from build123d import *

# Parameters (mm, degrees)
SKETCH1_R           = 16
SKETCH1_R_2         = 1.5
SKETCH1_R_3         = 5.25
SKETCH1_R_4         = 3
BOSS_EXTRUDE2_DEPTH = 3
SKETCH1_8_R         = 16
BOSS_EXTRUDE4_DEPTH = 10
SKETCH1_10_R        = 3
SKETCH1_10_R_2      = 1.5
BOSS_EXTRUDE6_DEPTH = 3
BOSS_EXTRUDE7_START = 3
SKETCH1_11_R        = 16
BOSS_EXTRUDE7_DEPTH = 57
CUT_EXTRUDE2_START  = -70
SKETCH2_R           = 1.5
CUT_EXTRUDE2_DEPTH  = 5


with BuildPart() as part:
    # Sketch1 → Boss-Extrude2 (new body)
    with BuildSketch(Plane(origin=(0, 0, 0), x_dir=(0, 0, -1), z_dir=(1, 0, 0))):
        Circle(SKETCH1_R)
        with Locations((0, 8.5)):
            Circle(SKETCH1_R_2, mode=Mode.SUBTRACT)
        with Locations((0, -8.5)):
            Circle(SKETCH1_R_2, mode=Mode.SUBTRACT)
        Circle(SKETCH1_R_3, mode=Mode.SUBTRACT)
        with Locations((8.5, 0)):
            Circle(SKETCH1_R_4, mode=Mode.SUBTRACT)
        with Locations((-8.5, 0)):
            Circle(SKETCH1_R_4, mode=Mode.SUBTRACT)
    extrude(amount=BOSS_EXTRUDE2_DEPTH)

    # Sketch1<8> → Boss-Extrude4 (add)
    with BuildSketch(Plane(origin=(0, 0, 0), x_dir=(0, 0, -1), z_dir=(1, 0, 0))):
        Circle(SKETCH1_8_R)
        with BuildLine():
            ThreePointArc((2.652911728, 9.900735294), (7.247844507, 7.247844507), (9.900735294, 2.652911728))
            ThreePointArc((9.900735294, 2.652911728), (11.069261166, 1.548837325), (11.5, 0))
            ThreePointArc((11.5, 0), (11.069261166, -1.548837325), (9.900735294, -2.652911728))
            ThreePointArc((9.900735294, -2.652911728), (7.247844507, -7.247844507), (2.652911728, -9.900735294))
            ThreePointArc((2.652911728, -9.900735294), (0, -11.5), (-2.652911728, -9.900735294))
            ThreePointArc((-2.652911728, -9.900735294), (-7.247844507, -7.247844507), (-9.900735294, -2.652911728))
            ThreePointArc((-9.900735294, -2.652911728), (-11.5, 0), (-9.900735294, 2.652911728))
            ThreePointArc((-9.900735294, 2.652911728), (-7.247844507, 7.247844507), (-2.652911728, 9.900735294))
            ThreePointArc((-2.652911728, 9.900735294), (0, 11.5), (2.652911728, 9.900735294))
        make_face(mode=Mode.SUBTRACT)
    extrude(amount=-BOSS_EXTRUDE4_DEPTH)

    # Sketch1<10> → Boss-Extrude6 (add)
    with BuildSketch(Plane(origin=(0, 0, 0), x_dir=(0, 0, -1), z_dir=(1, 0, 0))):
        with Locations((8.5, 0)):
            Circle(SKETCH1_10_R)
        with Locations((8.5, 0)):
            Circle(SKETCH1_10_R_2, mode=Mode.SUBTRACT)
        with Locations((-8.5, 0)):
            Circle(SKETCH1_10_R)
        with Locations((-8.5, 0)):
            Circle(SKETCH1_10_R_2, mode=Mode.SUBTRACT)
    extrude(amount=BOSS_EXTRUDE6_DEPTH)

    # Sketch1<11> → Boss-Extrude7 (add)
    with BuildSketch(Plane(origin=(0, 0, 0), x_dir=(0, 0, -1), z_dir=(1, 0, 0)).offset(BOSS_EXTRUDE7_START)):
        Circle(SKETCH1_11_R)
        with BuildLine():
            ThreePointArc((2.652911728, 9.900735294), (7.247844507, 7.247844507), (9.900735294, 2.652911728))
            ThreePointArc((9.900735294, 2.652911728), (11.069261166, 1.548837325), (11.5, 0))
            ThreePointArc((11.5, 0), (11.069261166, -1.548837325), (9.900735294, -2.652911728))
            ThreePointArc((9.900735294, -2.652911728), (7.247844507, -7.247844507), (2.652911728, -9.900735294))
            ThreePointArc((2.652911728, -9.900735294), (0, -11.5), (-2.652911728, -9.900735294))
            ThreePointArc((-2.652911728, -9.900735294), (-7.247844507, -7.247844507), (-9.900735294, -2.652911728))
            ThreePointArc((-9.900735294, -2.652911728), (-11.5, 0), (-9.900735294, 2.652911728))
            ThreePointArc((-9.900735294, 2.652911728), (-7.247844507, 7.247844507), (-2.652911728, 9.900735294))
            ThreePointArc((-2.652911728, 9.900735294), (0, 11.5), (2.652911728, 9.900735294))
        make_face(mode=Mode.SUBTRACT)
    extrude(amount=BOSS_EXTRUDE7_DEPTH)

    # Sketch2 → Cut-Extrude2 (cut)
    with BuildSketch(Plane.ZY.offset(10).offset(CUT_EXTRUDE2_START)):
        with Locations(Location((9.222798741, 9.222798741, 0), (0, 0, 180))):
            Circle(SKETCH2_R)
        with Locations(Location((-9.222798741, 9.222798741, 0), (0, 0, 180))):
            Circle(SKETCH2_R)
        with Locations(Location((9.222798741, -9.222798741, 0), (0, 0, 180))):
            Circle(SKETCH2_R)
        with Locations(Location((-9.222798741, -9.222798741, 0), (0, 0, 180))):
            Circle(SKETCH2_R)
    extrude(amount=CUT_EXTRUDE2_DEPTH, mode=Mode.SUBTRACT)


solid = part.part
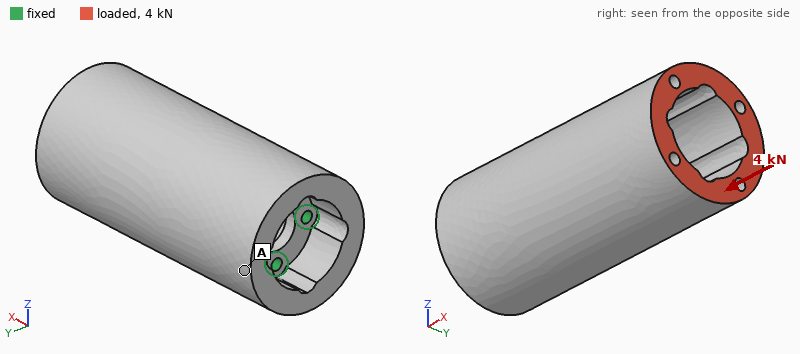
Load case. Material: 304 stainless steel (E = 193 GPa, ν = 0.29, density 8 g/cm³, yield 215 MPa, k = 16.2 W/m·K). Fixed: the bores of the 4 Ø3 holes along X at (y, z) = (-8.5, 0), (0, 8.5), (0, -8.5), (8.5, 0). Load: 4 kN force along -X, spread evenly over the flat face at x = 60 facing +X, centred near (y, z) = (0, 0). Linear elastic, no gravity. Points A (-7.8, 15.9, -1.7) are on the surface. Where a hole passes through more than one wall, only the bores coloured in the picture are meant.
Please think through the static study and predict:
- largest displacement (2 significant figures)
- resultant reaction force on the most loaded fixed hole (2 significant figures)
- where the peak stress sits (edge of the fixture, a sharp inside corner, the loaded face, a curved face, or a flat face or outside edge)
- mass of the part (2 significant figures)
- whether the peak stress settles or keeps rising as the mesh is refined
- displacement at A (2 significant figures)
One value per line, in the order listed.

4.5 µm
1.0 kN
edge of the fixture
260 g
keeps rising
1.7 µm
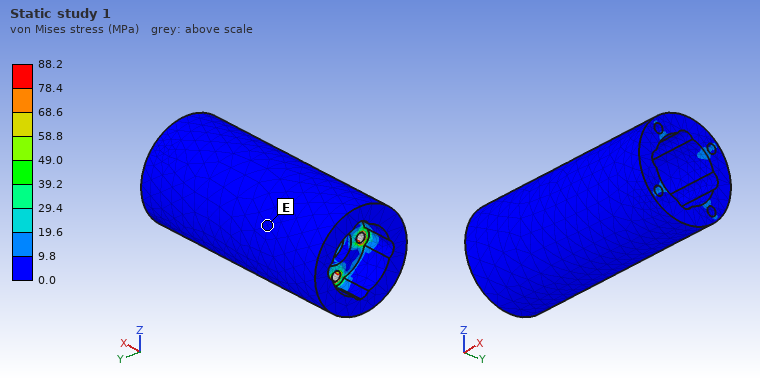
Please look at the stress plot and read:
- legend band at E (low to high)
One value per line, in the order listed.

0.0 to 9.8 MPa
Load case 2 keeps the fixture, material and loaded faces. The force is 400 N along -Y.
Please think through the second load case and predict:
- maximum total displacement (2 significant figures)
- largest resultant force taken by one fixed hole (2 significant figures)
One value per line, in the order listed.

17 µm
1.1 kN
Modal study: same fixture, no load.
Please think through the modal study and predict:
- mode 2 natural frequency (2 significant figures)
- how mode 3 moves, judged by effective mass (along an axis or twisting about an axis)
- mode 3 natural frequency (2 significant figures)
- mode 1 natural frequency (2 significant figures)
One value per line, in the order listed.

2900 Hz
twisting about X
10 kHz
2900 Hz
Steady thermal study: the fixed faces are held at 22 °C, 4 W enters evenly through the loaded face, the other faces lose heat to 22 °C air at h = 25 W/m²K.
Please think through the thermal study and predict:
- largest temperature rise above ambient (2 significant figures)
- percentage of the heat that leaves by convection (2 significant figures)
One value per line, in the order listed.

21 K
64 %
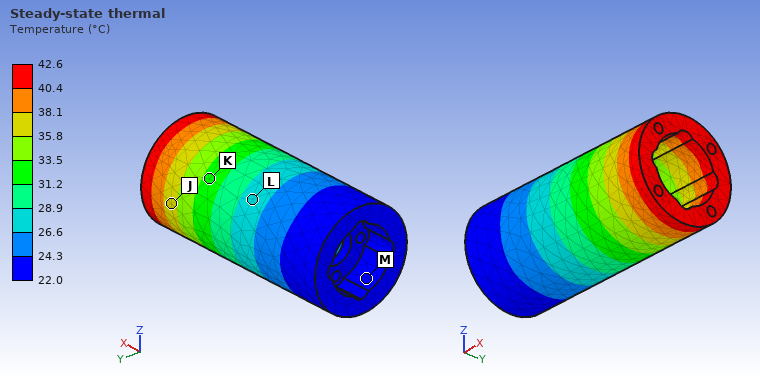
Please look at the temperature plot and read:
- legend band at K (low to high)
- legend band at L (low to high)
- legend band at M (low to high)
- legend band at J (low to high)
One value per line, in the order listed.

31.2 to 33.5 °C
26.6 to 28.9 °C
22.0 to 24.3 °C
35.8 to 38.1 °C
